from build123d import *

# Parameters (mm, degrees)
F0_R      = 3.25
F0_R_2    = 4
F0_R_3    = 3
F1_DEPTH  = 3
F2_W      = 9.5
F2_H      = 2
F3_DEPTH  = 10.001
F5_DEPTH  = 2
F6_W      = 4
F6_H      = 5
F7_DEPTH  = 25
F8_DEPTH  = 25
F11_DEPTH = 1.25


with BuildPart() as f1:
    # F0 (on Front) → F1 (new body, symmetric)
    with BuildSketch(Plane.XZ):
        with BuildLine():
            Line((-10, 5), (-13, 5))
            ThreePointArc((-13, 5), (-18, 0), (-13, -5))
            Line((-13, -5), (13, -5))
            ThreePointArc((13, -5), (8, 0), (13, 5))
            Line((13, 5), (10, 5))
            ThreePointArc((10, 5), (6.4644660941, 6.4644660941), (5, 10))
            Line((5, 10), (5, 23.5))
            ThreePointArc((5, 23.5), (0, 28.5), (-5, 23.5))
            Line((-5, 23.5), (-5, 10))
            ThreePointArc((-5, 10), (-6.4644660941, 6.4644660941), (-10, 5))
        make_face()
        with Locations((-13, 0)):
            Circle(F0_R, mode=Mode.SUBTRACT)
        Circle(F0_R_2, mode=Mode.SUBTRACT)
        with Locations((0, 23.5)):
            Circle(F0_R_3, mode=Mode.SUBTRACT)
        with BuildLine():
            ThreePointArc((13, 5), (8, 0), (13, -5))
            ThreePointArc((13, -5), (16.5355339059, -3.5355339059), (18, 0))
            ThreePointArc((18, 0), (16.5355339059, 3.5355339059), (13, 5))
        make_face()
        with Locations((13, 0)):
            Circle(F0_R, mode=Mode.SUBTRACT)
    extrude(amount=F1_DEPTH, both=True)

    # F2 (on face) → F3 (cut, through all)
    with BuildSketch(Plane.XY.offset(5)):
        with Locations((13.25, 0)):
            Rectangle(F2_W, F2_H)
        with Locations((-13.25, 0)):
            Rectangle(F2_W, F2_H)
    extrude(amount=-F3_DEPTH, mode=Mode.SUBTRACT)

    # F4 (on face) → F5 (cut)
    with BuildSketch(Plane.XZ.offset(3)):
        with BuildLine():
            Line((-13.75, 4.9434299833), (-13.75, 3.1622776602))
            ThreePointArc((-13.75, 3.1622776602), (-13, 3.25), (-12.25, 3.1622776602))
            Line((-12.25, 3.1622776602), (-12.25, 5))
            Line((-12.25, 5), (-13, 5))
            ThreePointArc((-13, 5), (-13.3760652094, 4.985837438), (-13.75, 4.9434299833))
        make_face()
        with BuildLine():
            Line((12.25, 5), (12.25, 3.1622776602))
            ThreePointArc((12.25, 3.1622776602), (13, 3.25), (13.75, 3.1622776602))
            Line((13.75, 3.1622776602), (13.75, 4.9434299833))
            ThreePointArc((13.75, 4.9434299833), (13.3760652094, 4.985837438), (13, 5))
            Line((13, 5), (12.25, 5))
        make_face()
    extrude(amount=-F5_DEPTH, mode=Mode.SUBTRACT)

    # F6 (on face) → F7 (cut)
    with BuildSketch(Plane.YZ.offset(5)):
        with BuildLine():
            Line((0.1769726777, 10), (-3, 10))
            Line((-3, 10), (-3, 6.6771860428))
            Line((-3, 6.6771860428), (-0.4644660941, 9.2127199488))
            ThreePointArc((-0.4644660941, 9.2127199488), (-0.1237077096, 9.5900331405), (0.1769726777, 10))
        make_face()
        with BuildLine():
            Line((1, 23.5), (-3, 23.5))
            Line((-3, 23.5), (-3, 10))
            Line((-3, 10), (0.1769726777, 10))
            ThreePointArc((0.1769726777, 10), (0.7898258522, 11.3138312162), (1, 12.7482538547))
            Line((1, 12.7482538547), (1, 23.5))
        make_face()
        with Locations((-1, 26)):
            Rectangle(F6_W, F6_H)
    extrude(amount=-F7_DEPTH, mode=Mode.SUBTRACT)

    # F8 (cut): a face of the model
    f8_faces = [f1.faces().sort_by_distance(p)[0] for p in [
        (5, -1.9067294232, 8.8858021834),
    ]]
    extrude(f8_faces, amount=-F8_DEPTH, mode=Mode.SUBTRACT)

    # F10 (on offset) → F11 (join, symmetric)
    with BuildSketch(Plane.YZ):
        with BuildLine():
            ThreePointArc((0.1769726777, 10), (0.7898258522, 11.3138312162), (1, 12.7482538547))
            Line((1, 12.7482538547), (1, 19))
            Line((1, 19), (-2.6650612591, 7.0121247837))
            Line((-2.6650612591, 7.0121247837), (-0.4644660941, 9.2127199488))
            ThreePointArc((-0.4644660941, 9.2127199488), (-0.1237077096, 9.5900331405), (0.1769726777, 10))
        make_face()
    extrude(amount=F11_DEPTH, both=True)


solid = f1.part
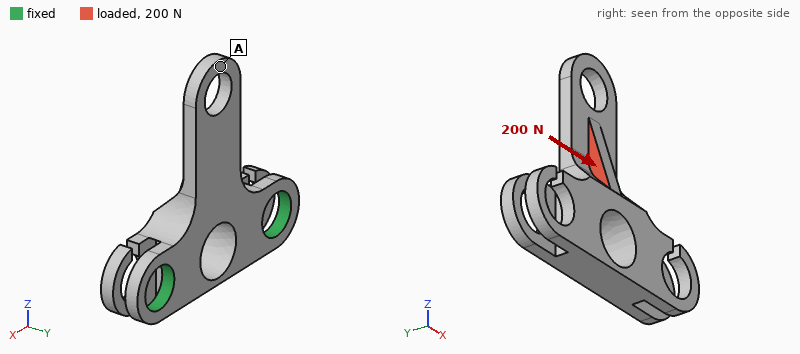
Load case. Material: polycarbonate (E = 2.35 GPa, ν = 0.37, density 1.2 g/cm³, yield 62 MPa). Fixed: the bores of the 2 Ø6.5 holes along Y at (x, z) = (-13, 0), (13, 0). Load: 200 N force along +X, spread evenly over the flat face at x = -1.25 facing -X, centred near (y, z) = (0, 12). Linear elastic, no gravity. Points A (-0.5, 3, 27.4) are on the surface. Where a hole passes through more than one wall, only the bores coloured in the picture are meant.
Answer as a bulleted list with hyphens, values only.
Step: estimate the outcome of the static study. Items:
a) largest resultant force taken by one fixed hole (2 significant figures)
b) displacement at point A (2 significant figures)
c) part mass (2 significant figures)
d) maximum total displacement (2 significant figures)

- 160 N
- 0.29 mm
- 2.1 g
- 0.36 mm
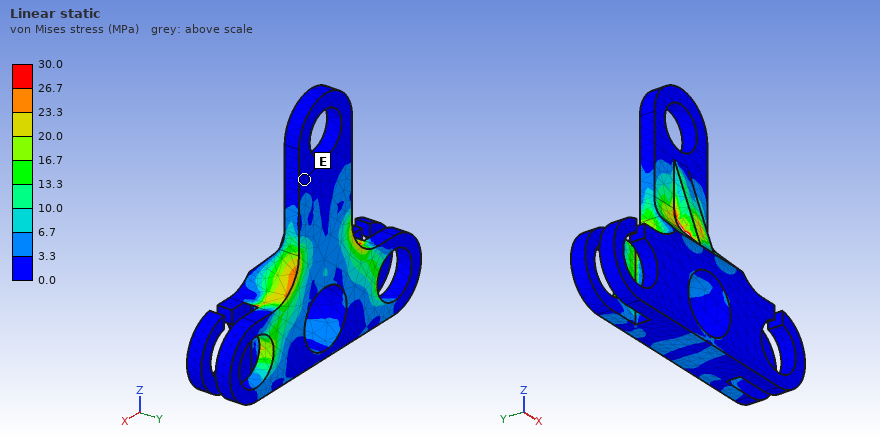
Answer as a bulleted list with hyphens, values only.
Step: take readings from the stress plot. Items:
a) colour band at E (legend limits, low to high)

- 0.0 to 3.3 MPa
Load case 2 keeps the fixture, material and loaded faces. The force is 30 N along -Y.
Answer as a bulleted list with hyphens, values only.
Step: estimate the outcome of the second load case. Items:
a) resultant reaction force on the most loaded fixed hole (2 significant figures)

- 25 N
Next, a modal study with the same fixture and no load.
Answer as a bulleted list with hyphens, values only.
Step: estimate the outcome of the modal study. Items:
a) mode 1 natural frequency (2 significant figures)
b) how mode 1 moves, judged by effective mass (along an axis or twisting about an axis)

- 1600 Hz
- along Y
